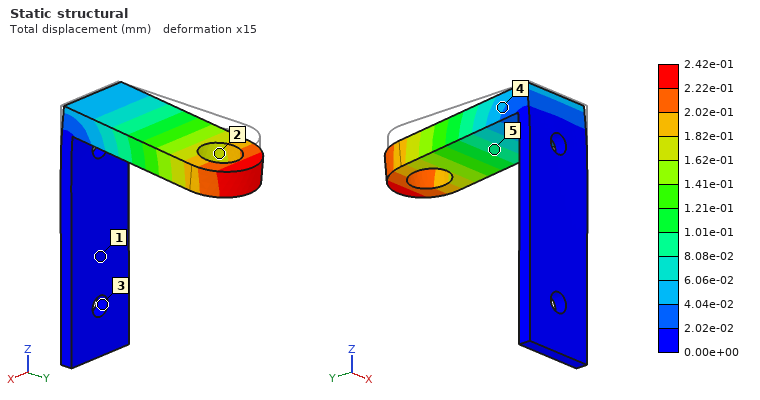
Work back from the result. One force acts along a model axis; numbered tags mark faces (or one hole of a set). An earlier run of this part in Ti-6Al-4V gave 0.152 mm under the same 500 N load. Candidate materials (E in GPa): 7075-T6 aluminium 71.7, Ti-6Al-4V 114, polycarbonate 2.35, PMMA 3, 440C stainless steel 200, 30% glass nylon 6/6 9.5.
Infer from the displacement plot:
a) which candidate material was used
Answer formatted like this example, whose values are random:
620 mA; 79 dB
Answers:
7075-T6 aluminium
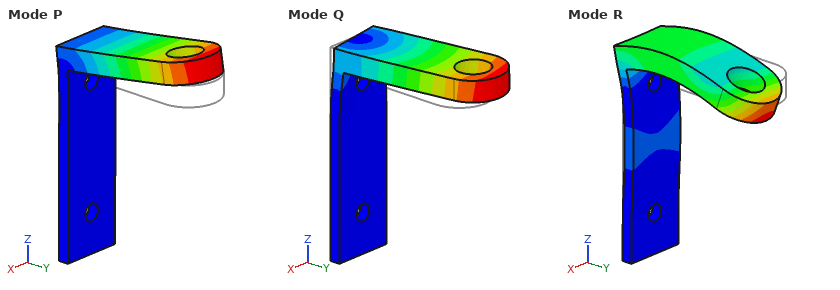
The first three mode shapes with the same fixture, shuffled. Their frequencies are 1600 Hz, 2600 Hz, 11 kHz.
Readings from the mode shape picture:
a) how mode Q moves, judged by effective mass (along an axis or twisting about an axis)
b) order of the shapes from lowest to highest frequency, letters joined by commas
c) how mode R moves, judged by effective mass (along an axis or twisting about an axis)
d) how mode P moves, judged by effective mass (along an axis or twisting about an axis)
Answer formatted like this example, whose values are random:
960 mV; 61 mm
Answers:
along X; P, Q, R; along Y; along Z
